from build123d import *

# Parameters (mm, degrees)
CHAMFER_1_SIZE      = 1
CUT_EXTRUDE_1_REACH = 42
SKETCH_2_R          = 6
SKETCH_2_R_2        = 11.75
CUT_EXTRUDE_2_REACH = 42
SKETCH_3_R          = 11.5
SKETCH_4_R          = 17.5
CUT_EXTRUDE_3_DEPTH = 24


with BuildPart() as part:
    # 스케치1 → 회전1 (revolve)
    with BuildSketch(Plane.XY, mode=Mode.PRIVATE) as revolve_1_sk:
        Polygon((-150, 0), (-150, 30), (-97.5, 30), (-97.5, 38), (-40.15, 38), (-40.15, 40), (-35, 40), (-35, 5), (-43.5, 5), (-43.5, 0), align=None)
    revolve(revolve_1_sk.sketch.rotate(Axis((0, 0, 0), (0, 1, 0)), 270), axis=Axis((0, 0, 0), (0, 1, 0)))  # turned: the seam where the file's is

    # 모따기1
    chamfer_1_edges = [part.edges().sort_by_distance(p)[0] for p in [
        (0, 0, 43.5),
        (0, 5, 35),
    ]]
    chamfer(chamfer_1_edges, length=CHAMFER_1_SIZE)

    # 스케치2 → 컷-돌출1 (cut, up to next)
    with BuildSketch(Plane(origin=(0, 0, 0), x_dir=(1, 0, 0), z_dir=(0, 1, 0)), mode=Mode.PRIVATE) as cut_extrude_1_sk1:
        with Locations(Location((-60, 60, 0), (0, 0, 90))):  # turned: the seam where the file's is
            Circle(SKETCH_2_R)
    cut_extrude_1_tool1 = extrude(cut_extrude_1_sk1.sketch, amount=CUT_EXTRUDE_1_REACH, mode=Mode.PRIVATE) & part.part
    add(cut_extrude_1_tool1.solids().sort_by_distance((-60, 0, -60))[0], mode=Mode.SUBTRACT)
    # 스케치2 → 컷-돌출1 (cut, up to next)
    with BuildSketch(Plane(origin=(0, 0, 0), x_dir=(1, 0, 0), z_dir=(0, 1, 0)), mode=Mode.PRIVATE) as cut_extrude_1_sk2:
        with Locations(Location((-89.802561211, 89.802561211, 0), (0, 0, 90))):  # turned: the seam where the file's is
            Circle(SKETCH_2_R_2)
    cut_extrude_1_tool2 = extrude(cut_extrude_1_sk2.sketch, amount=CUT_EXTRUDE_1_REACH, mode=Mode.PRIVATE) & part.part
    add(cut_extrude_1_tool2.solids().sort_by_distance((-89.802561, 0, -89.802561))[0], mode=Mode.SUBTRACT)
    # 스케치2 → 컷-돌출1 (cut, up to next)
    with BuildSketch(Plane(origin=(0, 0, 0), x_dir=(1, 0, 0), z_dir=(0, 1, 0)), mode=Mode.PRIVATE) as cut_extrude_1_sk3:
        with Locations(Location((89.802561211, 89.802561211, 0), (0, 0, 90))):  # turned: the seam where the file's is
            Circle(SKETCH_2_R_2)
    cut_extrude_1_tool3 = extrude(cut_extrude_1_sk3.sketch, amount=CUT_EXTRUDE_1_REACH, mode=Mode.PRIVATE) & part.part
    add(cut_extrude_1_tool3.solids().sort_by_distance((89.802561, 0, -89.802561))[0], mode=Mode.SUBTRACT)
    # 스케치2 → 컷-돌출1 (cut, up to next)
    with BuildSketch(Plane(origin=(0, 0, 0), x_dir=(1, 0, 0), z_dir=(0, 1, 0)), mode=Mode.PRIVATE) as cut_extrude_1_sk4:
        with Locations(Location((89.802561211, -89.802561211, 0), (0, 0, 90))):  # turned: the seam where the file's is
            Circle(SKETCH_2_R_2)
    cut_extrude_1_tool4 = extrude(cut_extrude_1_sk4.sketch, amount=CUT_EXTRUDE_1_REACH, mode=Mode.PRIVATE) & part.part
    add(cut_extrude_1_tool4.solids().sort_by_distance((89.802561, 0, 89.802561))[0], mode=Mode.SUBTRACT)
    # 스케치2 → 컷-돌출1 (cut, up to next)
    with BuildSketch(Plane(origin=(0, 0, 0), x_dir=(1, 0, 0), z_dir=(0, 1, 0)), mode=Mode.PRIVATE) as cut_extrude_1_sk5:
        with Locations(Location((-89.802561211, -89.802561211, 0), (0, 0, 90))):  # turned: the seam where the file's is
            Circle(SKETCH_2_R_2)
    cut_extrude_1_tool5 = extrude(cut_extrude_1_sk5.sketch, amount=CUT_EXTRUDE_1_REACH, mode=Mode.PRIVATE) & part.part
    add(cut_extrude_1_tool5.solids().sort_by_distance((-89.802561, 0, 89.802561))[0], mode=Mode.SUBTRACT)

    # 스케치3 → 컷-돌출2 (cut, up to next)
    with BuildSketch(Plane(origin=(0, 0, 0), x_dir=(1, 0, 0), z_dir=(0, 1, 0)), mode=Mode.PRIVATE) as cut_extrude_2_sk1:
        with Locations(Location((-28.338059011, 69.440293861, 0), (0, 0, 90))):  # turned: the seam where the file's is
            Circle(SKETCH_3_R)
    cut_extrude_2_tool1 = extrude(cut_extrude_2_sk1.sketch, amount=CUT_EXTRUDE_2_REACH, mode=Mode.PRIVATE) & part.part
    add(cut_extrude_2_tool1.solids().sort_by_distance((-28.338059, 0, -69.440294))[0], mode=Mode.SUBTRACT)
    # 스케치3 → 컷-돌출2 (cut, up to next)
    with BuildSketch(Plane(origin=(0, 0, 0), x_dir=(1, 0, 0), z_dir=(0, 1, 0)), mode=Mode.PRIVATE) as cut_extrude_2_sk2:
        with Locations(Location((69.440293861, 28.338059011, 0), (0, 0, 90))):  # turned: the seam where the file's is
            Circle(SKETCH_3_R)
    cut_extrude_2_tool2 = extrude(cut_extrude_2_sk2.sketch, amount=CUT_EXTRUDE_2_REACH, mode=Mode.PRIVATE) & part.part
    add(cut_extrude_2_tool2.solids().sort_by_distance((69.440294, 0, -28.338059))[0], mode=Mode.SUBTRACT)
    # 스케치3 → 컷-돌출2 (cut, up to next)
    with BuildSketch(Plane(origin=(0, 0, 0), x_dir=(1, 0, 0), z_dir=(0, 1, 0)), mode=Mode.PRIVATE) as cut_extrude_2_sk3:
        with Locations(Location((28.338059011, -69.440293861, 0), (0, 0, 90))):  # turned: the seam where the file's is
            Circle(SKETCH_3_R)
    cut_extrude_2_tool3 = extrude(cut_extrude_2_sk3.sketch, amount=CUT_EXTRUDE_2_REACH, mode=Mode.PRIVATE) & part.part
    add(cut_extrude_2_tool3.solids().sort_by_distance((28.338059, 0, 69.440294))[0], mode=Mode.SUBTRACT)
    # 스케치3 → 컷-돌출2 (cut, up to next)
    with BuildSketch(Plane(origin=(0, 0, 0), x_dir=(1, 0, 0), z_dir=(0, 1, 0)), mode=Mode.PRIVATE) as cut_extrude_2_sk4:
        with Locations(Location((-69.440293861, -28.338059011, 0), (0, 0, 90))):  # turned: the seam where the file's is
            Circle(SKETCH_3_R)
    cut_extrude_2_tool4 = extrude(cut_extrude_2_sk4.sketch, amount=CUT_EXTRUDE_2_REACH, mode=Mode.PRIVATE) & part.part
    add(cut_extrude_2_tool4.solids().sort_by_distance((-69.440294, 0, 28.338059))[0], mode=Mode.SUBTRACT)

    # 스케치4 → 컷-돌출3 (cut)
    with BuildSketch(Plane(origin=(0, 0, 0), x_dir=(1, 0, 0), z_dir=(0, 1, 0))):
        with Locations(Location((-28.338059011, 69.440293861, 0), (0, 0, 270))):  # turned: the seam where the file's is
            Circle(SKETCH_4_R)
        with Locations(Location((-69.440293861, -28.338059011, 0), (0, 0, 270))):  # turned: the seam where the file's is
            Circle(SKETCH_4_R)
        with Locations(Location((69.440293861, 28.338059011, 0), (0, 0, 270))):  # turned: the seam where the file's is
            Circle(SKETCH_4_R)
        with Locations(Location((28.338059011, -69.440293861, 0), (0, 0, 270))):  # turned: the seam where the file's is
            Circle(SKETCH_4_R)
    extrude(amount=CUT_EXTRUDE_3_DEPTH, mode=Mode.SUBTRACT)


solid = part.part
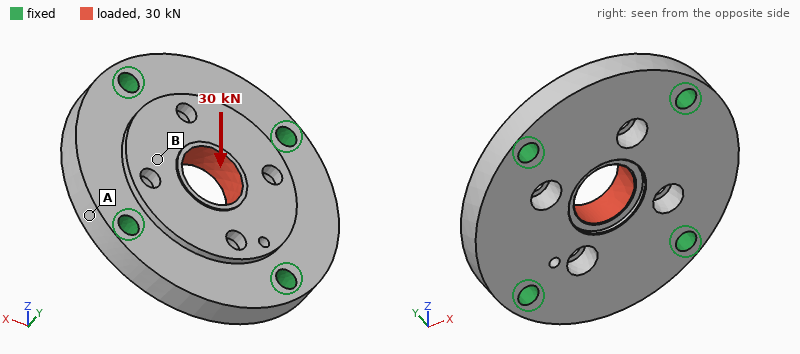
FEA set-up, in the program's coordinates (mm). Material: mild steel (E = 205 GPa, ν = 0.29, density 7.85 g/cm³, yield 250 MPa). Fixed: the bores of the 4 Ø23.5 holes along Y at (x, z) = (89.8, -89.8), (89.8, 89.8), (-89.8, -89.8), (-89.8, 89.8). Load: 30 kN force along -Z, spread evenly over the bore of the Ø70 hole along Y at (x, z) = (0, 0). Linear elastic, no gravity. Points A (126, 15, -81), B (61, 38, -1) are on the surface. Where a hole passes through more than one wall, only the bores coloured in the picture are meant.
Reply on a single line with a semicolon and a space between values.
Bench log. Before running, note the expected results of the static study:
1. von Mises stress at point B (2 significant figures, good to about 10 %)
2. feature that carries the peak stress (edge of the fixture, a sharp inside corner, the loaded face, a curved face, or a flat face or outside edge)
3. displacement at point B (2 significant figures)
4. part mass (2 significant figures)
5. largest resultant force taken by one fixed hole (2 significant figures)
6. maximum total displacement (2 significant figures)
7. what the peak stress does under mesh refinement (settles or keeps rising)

3.4 MPa; edge of the fixture; 1.4 µm; 16 kg; 8.2 kN; 3.3 µm; keeps rising
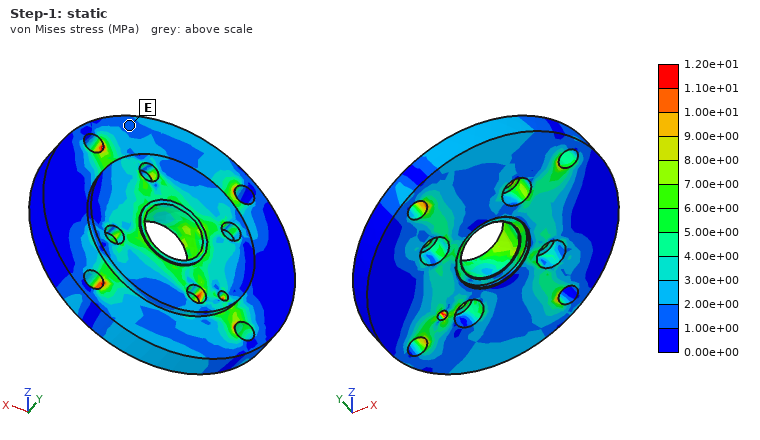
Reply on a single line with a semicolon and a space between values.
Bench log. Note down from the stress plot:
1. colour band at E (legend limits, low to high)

1.00e+00 to 2.00e+00 MPa
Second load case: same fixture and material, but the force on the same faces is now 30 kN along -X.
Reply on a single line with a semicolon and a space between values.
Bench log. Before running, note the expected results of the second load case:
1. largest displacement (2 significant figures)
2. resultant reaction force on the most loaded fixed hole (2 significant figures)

3.2 µm; 8.3 kN
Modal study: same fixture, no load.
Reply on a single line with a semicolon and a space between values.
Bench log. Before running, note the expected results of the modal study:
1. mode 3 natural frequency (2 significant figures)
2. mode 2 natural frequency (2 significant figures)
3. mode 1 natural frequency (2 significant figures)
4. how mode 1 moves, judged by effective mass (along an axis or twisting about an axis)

3900 Hz; 3700 Hz; 3500 Hz; along Y
